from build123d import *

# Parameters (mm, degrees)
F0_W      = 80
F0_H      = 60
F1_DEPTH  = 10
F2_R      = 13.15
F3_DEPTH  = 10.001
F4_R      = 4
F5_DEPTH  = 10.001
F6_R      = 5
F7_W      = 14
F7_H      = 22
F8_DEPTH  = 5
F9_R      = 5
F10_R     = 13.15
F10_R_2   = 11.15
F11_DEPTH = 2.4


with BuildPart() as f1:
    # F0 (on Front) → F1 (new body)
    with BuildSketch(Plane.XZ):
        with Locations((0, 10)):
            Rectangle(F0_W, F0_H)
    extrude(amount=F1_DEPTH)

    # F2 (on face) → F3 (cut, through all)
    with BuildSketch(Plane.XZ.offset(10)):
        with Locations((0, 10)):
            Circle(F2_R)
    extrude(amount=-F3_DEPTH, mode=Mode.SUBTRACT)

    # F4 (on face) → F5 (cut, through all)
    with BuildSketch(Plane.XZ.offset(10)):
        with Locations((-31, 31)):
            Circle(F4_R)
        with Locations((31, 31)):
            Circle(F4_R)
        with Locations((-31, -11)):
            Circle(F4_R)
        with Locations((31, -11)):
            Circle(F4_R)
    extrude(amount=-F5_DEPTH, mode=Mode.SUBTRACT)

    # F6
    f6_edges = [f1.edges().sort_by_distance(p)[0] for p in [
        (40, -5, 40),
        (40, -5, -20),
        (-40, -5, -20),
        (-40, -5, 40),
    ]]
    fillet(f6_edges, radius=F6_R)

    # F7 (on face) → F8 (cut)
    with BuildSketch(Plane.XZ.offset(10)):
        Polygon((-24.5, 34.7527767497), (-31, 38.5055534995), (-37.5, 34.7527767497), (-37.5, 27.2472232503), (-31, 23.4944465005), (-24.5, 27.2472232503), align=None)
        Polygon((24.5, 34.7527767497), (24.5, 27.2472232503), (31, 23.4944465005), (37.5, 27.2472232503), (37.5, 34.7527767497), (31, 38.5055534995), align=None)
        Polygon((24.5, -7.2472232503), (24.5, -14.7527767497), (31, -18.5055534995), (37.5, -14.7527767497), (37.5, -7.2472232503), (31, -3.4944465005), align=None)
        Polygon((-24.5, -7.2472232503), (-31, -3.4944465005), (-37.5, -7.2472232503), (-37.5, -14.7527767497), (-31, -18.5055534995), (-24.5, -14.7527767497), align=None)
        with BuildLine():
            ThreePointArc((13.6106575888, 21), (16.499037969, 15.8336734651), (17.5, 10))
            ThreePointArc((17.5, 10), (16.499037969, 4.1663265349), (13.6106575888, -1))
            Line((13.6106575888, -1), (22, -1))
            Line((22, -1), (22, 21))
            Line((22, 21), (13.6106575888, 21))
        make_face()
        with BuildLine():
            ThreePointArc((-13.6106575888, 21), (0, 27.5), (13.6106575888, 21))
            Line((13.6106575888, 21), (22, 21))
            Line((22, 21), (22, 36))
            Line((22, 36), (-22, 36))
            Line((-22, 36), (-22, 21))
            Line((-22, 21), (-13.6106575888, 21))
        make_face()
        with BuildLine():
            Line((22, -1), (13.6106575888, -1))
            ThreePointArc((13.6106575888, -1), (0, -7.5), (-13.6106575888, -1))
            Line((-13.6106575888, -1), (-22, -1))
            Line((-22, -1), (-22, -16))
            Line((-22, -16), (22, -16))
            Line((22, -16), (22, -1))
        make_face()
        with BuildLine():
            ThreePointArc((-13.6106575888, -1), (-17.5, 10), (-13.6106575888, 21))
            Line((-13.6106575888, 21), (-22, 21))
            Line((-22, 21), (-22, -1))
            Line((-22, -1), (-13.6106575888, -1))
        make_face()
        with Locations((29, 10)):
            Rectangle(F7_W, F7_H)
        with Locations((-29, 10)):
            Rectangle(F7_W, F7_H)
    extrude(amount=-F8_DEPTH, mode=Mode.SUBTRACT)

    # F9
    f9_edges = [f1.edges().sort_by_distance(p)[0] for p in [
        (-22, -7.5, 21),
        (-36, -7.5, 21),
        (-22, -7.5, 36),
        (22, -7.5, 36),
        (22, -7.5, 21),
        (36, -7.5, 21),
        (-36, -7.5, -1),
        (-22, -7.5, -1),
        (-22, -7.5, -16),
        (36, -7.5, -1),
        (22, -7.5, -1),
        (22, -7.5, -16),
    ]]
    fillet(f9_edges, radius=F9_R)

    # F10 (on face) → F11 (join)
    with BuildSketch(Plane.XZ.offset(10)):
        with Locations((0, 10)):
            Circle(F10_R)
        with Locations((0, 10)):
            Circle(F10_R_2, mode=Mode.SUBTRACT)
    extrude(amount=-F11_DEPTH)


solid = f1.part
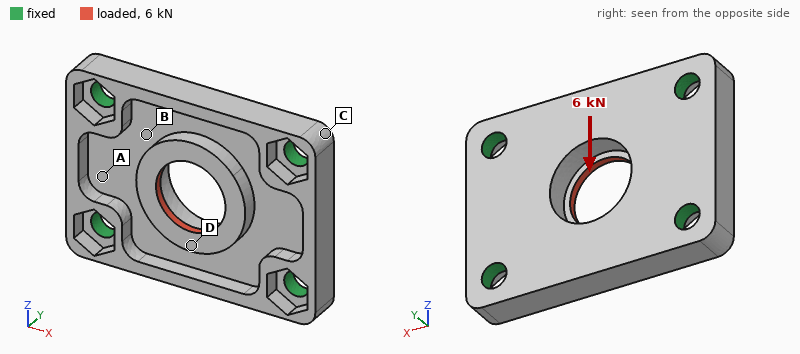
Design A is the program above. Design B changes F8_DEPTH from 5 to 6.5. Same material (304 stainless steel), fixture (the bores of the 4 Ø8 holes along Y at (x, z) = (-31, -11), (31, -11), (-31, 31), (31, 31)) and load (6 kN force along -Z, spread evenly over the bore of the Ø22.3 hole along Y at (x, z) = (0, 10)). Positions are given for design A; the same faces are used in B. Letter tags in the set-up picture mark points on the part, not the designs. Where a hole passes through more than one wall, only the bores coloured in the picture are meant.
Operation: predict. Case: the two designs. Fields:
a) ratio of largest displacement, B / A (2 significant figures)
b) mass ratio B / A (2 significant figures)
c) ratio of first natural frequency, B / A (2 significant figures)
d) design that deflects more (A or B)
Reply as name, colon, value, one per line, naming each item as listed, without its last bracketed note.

ratio of largest displacement, B / A: 1.8
mass ratio B / A: 0.88
ratio of first natural frequency, B / A: 0.85
design that deflects more: B
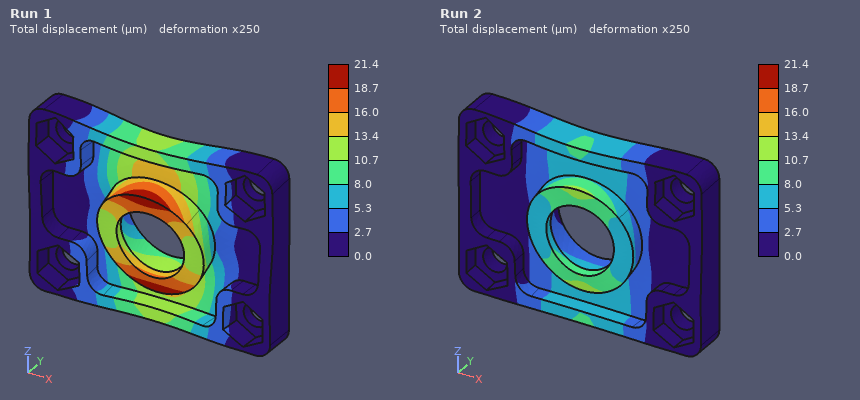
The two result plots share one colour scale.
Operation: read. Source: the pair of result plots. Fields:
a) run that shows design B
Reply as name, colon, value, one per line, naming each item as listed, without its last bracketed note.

run that shows design B: Run 1
